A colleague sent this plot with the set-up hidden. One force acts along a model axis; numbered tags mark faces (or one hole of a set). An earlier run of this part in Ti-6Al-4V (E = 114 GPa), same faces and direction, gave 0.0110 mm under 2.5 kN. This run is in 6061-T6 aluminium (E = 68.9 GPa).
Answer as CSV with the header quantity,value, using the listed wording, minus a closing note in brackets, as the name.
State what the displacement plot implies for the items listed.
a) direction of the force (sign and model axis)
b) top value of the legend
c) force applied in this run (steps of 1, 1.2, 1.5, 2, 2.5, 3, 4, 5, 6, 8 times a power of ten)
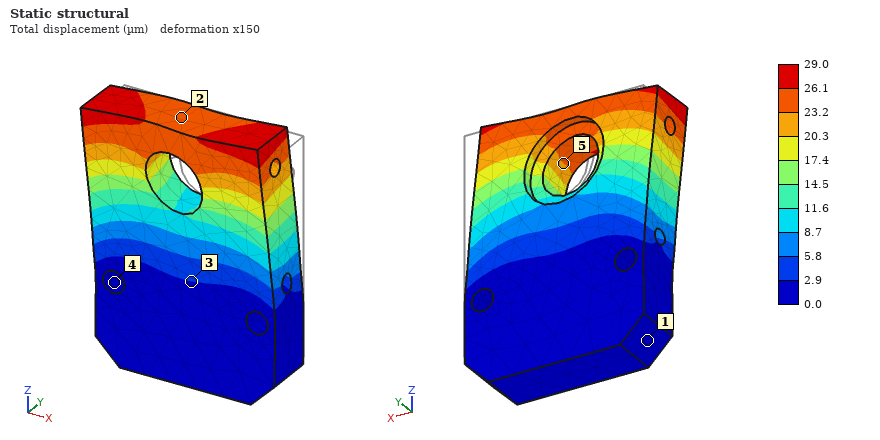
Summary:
quantity,value
direction of the force,-X
top value of the legend,29.0 µm
force applied in this run,4 kN
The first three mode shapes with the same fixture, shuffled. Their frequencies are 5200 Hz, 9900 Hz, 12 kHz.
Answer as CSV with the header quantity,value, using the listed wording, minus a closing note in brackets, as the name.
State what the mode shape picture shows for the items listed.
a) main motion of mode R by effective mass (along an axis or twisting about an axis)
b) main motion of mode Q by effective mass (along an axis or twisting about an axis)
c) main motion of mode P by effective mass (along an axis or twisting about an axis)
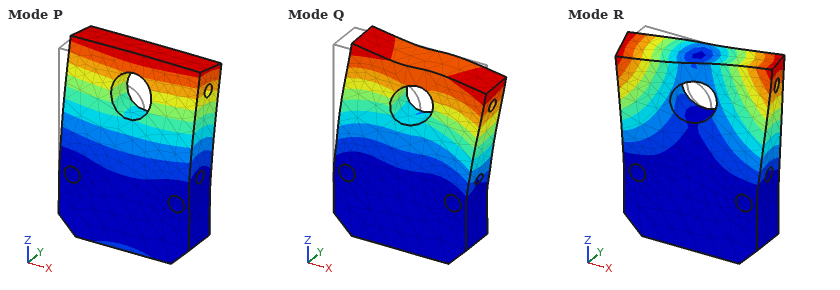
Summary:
quantity,value
main motion of mode R by effective mass,twisting about Z
main motion of mode Q by effective mass,along X
main motion of mode P by effective mass,along Y
